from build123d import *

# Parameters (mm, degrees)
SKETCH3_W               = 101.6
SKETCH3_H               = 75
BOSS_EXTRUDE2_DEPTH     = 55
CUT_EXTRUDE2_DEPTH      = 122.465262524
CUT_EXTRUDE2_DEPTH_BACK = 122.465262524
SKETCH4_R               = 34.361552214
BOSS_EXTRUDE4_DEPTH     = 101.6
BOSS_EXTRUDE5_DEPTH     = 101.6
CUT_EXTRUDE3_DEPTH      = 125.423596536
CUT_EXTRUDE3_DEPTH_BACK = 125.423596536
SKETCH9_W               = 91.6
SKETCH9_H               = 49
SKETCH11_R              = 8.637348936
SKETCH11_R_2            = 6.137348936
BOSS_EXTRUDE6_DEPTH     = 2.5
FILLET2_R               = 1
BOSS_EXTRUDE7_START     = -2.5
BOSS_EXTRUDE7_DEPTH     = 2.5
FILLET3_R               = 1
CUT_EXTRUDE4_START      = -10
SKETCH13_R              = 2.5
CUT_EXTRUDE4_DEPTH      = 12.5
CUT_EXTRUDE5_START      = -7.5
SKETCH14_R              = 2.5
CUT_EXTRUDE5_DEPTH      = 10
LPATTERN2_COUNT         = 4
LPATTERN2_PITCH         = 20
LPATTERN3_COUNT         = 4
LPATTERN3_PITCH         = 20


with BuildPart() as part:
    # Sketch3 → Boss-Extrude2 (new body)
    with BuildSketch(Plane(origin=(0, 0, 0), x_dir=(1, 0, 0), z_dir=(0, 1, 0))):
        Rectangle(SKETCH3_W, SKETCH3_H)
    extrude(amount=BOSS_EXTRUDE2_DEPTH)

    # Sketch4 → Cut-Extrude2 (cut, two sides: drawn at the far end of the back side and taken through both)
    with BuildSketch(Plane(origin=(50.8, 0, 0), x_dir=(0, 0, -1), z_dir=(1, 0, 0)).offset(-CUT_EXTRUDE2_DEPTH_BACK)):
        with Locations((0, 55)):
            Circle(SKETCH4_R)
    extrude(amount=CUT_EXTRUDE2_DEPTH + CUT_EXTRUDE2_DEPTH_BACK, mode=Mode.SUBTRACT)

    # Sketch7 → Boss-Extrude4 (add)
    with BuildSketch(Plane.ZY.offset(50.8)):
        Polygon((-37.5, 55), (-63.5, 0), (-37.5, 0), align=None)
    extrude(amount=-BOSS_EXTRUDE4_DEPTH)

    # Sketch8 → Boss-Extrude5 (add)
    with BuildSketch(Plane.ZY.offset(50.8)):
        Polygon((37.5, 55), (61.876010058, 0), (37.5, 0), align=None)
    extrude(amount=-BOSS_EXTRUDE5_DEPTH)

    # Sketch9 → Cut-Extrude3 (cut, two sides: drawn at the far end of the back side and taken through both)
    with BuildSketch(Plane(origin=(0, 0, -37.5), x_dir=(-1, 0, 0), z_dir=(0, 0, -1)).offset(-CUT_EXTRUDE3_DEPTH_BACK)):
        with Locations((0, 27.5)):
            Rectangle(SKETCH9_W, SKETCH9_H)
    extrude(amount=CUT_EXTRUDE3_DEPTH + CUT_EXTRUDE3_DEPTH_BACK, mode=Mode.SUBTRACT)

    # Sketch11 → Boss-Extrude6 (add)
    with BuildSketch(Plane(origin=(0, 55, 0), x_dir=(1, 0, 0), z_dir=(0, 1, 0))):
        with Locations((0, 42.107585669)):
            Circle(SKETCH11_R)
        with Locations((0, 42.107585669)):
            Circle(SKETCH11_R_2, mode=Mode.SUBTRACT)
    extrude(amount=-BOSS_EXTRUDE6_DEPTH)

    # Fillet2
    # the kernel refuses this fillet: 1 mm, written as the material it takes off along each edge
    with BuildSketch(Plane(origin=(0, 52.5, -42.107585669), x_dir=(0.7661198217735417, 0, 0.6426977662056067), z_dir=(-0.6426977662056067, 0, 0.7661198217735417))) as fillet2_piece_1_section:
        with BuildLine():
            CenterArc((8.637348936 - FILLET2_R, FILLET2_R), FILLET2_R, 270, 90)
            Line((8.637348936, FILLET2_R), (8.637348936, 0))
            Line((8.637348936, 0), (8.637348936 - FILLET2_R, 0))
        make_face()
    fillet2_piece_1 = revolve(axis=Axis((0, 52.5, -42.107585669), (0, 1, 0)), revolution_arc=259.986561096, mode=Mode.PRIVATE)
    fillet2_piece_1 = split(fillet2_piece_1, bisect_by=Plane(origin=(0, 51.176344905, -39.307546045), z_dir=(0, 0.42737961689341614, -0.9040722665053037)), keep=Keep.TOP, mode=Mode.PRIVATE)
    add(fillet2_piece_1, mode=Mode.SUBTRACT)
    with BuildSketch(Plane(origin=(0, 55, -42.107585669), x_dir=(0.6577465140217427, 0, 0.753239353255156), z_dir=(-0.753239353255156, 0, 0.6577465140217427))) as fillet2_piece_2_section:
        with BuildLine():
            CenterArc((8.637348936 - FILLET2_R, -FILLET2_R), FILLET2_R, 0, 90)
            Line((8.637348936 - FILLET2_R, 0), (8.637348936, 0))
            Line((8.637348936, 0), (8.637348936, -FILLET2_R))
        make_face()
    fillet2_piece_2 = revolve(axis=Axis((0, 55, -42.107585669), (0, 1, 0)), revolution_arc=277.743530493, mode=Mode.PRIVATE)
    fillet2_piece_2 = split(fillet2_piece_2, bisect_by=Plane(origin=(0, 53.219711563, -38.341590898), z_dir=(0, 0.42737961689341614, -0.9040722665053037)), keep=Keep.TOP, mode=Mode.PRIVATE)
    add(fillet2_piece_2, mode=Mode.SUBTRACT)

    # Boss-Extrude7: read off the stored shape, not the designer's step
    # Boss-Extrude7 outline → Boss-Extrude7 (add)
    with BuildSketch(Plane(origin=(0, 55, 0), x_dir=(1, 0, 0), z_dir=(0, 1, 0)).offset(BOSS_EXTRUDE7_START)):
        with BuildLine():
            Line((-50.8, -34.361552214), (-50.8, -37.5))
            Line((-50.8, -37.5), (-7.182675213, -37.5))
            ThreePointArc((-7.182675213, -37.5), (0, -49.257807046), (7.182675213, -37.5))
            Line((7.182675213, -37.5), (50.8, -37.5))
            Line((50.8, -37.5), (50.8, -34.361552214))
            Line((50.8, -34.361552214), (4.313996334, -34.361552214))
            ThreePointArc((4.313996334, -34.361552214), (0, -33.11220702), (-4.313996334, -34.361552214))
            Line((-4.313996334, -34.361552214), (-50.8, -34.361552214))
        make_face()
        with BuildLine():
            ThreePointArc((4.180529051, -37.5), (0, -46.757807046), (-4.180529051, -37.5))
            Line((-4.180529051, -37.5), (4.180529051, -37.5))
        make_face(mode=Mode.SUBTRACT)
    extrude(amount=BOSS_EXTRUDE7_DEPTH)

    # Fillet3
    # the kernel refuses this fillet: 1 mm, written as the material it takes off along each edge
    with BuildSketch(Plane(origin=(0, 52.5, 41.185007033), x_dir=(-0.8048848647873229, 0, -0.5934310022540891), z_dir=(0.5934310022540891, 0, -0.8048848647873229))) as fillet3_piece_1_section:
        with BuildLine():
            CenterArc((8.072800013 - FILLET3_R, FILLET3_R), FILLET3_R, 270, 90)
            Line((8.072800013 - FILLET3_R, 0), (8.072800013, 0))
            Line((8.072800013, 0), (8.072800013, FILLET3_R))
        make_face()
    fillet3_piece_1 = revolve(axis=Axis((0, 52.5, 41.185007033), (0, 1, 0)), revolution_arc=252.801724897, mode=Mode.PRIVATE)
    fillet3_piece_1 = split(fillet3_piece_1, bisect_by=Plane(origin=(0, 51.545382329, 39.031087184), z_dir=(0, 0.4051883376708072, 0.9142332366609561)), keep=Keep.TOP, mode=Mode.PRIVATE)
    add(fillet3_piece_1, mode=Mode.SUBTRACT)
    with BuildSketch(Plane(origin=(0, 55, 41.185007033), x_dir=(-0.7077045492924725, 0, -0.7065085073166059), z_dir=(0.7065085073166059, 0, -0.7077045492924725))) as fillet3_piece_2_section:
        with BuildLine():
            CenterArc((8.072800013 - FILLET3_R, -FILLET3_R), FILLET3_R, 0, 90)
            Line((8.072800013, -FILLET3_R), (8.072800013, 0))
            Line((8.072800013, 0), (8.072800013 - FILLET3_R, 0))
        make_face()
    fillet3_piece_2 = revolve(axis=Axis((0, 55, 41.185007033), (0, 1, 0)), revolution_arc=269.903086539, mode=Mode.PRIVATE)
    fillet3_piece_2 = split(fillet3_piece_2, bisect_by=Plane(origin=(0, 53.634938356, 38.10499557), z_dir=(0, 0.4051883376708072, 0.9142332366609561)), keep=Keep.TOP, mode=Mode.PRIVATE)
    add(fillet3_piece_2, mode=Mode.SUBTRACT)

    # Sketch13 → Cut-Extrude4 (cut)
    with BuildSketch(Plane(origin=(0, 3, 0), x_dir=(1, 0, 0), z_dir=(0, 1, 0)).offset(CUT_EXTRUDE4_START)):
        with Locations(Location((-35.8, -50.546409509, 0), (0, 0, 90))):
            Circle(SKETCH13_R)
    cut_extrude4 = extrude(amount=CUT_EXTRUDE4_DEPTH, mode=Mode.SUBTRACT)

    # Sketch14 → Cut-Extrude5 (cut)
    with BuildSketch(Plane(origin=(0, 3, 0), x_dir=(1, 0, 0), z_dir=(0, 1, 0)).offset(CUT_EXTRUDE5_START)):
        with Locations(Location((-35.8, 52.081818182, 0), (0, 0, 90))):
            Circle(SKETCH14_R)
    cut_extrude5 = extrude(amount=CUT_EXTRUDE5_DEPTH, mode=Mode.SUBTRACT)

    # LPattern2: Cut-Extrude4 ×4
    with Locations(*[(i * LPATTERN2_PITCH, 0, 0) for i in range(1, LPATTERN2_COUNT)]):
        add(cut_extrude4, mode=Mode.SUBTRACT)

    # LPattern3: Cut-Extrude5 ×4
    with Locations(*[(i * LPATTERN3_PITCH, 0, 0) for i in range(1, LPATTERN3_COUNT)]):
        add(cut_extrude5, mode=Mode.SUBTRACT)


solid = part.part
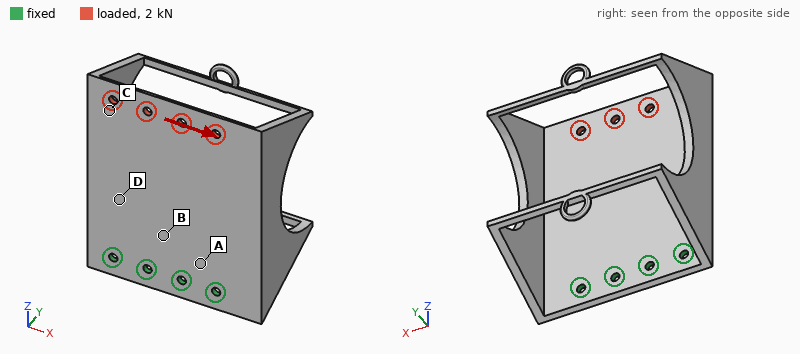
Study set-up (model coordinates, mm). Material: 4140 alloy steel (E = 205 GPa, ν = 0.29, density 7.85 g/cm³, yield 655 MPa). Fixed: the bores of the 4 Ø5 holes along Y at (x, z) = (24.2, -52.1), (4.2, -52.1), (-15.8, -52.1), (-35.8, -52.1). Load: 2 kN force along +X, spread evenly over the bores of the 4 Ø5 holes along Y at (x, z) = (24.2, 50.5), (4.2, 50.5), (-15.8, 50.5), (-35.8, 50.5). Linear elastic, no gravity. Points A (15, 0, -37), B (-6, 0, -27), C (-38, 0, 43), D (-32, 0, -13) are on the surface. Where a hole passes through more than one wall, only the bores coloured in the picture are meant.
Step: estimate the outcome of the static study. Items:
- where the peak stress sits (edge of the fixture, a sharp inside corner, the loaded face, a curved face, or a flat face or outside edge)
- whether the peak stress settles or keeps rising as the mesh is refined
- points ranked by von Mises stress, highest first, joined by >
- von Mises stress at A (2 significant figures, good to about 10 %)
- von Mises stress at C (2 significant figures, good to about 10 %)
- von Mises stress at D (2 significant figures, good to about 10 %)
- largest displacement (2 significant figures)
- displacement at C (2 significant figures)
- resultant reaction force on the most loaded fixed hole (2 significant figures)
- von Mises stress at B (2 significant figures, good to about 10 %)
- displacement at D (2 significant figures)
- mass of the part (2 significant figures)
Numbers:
edge of the fixture
keeps rising
A > B > D > C
33 MPa
9.5 MPa
19 MPa
42 µm
33 µm
3.1 kN
26 MPa
12 µm
570 g
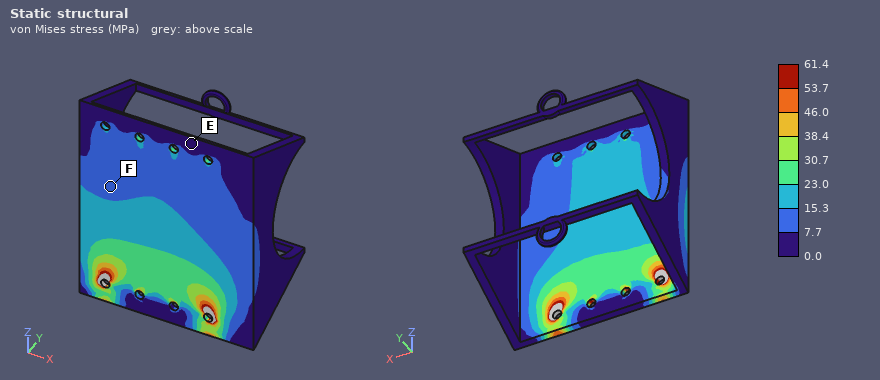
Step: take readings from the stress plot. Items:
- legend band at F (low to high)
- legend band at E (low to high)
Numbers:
7.7 to 15.3 MPa
0.0 to 7.7 MPa
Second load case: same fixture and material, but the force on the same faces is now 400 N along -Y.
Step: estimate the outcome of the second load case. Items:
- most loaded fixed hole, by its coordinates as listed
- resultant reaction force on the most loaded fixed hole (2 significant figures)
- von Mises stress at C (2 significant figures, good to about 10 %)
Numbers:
(-15.8, -52.1)
310 N
32 MPa
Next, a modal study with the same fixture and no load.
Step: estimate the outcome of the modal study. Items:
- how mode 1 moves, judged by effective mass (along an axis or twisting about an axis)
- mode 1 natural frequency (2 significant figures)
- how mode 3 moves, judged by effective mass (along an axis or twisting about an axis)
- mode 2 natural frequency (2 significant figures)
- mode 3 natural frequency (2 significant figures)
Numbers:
along Y
230 Hz
along X
360 Hz
1000 Hz
